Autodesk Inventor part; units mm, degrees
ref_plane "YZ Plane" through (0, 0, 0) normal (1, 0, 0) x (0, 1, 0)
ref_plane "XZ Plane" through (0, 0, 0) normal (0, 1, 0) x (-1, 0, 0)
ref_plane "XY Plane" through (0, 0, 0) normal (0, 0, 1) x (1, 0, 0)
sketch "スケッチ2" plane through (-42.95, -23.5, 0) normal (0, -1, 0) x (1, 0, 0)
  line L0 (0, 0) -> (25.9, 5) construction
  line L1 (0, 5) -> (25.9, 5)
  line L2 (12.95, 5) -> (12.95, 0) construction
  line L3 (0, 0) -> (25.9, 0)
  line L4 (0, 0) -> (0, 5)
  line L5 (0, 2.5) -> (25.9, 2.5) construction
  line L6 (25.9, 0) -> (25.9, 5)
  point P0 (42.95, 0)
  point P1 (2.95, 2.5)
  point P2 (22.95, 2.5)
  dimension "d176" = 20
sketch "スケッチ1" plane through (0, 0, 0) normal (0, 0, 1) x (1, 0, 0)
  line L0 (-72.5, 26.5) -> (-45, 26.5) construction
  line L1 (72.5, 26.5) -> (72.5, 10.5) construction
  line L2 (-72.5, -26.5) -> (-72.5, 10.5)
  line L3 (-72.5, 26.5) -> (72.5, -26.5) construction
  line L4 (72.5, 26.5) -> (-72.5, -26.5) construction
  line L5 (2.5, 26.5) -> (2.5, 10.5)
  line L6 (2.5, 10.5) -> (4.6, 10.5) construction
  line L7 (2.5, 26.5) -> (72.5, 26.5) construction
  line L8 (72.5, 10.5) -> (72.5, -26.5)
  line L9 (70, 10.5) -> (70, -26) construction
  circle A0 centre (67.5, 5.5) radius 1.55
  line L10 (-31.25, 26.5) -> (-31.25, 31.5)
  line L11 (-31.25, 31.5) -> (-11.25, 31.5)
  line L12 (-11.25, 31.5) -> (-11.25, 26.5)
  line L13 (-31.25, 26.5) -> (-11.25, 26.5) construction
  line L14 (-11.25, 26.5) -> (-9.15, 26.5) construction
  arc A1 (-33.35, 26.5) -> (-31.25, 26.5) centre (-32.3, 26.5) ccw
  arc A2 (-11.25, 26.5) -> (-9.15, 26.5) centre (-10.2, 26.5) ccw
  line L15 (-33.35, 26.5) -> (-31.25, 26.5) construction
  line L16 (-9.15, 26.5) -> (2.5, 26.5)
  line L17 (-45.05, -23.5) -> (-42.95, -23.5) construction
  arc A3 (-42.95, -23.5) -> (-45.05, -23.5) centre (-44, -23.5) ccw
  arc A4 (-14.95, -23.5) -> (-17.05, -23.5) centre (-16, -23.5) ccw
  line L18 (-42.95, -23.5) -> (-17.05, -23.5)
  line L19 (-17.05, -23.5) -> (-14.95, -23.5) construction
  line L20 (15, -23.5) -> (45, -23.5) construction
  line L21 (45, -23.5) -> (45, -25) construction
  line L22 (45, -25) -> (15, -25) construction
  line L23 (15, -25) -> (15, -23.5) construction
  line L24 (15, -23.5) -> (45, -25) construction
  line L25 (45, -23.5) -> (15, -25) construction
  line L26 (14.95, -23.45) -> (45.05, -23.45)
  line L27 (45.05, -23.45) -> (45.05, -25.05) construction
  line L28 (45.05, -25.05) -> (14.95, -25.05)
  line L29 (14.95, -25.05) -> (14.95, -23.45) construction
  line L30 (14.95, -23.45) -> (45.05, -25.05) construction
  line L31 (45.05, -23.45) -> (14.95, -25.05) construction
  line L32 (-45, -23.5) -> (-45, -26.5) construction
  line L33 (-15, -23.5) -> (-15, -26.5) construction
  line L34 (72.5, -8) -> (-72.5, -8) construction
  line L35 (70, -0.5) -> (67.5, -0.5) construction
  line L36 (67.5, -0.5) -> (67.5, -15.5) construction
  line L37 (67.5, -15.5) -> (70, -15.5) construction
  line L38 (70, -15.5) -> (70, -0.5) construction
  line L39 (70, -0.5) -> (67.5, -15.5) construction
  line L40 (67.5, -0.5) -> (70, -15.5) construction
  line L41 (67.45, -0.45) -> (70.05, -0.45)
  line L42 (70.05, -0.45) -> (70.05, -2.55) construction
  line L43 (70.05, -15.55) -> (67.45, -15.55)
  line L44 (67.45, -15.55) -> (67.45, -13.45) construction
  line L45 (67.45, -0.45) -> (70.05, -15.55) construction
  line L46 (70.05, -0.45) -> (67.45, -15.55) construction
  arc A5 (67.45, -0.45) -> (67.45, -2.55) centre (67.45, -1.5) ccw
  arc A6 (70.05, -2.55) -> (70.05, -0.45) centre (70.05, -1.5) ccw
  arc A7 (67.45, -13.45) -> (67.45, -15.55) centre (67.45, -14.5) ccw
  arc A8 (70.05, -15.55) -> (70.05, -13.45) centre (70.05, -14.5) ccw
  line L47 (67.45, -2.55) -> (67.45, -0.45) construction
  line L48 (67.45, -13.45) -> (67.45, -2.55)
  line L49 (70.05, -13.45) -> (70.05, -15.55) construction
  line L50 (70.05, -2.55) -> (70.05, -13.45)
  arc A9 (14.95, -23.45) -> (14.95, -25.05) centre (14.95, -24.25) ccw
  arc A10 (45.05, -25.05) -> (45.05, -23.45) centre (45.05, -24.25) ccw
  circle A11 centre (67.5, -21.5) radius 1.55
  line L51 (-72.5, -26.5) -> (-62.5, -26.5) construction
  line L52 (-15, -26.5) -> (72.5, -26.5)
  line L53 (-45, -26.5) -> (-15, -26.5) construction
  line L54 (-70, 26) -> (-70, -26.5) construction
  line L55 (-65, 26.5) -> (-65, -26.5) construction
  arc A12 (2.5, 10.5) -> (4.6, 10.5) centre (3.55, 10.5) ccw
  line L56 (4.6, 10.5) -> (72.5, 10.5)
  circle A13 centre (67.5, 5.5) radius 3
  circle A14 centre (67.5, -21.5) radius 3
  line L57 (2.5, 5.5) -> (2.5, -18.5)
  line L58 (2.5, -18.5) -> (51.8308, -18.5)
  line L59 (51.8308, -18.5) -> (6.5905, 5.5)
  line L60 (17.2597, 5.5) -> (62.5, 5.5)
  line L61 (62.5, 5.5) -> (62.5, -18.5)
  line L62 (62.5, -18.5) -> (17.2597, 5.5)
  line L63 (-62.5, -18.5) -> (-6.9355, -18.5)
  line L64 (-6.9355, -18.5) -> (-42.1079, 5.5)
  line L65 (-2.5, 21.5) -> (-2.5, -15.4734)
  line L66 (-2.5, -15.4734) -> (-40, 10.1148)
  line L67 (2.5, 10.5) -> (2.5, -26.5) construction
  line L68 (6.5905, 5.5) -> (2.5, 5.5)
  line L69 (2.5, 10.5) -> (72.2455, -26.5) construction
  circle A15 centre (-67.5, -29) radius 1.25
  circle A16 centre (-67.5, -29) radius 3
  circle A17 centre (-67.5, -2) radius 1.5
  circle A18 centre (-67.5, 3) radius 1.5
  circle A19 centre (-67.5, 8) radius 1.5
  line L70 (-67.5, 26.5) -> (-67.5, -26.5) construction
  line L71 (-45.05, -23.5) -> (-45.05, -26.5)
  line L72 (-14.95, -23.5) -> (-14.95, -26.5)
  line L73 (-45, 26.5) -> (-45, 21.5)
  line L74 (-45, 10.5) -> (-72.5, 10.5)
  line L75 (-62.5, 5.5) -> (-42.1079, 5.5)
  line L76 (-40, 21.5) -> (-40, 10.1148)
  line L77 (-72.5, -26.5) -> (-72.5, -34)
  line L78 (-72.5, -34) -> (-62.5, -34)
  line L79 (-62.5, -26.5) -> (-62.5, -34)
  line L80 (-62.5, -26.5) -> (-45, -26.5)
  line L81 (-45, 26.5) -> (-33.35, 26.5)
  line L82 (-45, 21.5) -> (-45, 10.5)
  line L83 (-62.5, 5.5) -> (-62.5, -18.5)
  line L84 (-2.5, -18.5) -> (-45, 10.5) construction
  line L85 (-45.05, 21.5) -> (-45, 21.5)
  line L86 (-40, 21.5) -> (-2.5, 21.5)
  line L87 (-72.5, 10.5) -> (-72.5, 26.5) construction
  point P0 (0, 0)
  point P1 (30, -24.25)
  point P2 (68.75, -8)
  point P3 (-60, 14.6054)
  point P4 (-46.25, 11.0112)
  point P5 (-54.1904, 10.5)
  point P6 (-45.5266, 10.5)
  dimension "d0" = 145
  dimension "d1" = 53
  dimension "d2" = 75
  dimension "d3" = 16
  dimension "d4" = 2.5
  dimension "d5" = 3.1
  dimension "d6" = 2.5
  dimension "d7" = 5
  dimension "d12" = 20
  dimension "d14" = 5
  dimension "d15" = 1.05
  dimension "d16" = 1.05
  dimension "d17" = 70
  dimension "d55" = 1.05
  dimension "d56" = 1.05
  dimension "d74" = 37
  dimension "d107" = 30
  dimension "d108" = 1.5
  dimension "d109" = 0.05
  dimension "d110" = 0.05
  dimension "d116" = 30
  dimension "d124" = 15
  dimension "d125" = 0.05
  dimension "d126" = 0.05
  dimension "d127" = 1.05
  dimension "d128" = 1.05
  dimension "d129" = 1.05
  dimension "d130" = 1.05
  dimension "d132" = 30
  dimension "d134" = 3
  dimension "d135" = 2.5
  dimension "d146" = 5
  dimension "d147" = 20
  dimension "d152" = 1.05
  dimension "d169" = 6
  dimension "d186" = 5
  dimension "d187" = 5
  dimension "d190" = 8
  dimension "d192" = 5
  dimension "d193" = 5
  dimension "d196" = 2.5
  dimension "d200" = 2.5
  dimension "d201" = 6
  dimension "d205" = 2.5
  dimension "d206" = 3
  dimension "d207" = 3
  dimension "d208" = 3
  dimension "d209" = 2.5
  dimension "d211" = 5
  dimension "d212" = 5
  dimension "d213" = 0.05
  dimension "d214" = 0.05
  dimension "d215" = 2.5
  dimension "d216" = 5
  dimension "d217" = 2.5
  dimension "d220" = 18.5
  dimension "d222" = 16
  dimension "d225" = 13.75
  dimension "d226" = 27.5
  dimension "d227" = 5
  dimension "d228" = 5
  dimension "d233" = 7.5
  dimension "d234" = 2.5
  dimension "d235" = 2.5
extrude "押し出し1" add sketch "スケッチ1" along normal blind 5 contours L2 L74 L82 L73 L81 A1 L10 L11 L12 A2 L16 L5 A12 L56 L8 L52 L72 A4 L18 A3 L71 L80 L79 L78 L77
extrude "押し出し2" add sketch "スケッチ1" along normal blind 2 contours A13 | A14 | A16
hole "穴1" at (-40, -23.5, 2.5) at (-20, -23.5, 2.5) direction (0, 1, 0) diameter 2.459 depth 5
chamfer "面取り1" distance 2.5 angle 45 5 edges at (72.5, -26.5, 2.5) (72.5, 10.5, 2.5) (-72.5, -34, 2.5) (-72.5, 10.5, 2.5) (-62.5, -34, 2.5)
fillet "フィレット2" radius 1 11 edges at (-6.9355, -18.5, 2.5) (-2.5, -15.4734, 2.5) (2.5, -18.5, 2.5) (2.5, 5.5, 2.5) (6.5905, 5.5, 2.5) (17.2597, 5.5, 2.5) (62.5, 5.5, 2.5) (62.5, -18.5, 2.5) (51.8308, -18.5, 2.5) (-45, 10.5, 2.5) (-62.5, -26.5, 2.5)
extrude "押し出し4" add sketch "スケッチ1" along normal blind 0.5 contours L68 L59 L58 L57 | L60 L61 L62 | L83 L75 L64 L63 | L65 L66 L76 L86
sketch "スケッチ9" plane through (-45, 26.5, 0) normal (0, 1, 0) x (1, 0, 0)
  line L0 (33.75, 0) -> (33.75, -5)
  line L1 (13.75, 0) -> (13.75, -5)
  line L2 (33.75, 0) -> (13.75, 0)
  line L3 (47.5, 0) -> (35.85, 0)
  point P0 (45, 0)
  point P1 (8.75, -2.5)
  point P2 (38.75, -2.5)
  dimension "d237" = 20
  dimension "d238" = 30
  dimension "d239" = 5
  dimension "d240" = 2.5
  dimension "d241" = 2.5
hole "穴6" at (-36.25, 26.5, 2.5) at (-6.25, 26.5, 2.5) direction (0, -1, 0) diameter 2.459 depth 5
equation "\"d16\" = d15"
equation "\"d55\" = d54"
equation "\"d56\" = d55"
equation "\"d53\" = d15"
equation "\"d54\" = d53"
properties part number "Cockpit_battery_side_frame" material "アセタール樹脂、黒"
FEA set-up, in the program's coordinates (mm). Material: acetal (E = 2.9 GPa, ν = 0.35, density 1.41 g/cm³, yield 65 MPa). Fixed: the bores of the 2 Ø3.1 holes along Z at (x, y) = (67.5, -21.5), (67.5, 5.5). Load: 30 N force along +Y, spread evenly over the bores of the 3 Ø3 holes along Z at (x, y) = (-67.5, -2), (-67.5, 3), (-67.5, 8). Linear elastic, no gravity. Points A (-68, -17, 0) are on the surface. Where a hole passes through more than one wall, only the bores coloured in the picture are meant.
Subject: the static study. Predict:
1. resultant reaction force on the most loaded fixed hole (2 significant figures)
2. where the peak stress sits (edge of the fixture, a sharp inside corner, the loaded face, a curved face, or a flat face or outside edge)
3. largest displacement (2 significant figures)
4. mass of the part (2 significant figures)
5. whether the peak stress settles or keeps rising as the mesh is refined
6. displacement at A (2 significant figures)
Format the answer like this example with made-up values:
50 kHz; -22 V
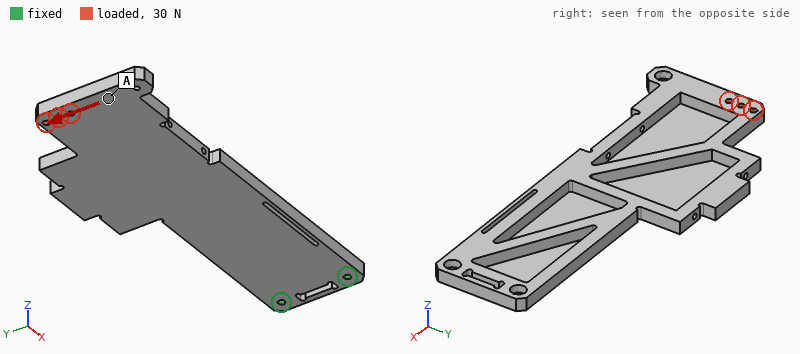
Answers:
140 N; edge of the fixture; 1.7 mm; 23 g; keeps rising; 1.4 mm
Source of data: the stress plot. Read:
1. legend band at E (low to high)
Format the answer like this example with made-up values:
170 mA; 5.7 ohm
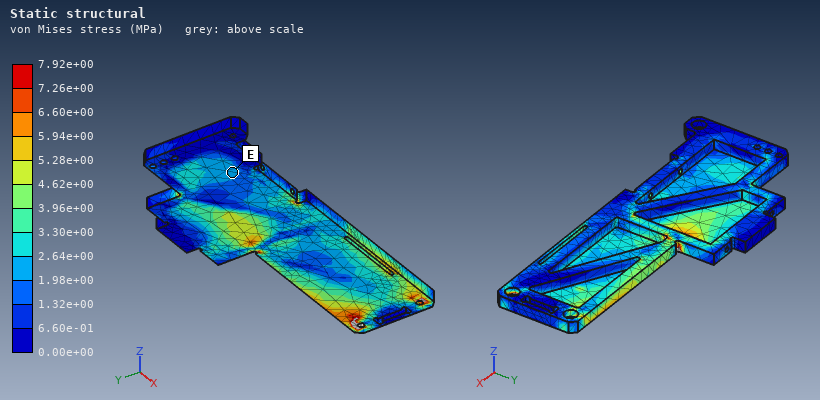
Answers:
1.98e+00 to 2.64e+00 MPa
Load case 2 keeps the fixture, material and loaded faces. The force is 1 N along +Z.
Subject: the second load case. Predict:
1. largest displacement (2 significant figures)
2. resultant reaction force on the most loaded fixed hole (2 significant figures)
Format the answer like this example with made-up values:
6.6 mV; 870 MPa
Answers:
1.9 mm; 2.5 N
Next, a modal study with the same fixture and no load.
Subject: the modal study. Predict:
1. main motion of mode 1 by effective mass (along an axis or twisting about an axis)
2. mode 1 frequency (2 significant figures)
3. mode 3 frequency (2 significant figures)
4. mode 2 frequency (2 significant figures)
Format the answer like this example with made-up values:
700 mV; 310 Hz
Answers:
along Z; 45 Hz; 290 Hz; 170 Hz
